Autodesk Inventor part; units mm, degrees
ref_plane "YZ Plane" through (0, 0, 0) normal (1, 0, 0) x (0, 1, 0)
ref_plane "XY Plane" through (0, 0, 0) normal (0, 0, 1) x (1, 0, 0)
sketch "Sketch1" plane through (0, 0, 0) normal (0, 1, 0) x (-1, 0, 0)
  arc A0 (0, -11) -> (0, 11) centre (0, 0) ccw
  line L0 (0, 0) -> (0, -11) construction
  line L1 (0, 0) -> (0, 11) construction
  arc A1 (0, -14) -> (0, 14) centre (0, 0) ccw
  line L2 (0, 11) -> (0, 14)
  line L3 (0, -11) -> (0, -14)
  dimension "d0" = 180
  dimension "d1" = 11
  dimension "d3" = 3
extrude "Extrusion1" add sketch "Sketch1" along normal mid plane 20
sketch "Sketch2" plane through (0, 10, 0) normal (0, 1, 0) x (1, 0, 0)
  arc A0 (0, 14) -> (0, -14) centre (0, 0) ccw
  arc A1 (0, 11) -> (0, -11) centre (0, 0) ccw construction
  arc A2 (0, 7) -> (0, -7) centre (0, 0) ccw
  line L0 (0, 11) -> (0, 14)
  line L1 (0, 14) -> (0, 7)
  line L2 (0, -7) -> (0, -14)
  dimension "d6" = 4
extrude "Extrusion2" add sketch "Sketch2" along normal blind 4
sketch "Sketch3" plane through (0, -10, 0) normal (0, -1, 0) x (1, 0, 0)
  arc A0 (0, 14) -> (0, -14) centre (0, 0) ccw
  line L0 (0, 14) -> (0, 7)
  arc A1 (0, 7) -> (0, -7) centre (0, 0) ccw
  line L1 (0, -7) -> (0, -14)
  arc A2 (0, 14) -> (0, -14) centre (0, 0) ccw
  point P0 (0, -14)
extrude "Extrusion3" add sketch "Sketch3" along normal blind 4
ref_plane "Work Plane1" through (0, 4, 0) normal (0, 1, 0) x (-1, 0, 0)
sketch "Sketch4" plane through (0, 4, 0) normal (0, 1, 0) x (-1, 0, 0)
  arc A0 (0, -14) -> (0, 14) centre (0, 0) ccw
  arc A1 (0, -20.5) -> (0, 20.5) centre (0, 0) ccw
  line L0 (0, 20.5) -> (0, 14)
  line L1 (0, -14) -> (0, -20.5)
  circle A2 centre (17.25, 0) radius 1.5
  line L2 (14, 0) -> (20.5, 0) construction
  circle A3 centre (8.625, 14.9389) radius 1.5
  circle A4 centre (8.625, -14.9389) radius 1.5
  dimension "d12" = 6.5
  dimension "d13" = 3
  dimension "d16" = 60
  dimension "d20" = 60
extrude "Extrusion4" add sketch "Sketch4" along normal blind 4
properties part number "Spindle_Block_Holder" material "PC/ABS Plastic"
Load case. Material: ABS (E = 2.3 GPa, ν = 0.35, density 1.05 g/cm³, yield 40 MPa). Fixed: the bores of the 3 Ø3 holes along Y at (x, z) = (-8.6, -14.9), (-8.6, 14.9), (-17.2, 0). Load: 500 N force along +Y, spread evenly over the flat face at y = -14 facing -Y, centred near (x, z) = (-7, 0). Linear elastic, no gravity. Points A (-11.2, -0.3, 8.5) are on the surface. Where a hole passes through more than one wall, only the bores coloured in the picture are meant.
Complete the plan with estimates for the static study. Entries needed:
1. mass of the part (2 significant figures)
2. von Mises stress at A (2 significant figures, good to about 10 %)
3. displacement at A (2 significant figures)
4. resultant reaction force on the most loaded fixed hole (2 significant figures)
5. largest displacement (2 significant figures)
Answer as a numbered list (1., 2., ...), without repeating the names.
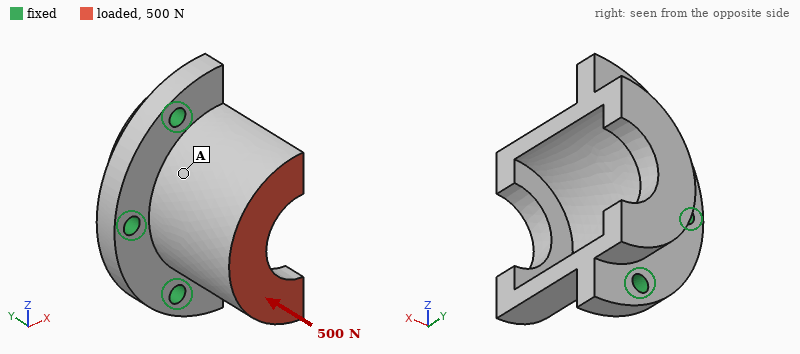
1. 5.8 g
2. 4.2 MPa
3. 0.053 mm
4. 220 N
5. 0.26 mm
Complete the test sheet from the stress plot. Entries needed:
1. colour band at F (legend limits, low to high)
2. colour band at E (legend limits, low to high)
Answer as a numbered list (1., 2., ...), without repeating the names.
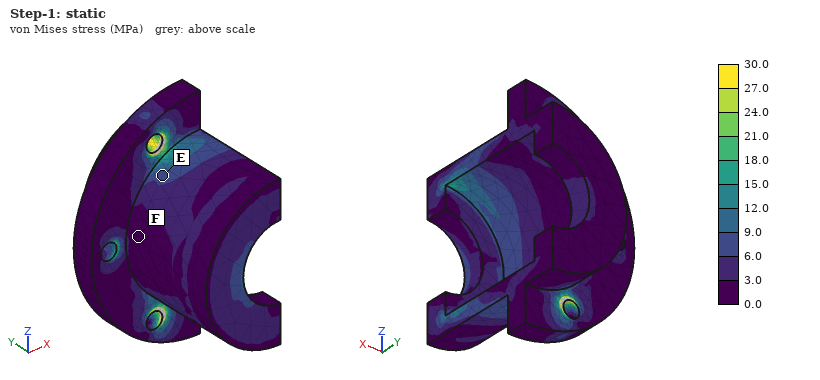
1. 0.0 to 3.0 MPa
2. 6.0 to 9.0 MPa
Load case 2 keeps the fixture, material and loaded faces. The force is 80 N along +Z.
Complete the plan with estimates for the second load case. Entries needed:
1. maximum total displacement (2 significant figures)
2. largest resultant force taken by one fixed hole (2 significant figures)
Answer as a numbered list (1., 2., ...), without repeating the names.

1. 0.25 mm
2. 63 N
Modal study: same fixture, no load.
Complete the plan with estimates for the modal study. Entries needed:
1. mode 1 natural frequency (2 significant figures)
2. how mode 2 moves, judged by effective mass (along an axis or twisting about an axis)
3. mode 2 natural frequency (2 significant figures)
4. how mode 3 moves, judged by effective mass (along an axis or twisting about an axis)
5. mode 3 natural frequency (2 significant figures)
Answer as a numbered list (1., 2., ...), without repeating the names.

1. 2700 Hz
2. along X
3. 2800 Hz
4. along Z
5. 5300 Hz
